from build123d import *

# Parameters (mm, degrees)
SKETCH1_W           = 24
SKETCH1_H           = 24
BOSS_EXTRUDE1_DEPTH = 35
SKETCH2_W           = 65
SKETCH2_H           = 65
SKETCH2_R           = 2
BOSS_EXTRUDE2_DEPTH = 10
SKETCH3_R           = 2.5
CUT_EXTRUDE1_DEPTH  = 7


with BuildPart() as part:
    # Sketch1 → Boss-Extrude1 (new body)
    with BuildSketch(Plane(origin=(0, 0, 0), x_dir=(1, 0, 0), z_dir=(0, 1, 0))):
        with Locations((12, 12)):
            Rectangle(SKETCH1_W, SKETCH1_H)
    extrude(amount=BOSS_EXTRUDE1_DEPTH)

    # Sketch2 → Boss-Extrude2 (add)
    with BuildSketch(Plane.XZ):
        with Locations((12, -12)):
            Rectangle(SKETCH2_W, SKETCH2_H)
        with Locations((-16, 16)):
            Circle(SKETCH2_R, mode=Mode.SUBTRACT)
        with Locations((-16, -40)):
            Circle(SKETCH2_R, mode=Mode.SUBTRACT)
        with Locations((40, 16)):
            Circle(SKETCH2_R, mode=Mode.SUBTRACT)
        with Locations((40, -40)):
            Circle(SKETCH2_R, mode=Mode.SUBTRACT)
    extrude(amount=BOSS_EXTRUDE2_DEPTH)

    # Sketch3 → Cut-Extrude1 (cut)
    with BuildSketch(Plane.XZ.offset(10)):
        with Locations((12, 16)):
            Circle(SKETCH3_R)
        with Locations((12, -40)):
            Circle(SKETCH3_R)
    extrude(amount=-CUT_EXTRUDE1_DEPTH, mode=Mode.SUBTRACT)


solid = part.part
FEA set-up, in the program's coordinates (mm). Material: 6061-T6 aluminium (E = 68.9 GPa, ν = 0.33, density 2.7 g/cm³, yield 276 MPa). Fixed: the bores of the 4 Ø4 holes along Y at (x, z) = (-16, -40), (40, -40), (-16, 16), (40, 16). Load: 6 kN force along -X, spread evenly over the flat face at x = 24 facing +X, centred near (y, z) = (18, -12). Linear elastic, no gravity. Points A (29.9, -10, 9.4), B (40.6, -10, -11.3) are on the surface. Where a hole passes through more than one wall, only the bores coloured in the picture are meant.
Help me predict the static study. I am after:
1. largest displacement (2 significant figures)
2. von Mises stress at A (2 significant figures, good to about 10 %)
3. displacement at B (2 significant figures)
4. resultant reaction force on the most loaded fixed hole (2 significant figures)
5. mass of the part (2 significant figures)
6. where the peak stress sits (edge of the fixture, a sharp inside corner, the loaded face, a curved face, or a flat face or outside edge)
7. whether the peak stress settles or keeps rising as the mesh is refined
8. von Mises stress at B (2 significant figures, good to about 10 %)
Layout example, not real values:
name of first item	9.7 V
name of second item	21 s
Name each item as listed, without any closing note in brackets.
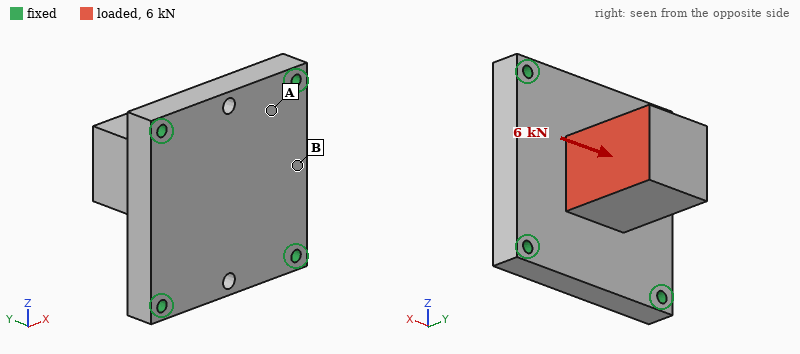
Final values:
largest displacement	94 µm
von Mises stress at A	9.9 MPa
displacement at B	20 µm
resultant reaction force on the most loaded fixed hole	2.2 kN
mass of the part	170 g
where the peak stress sits	edge of the fixture
whether the peak stress settles or keeps rising as the mesh is refined	keeps rising
von Mises stress at B	29 MPa
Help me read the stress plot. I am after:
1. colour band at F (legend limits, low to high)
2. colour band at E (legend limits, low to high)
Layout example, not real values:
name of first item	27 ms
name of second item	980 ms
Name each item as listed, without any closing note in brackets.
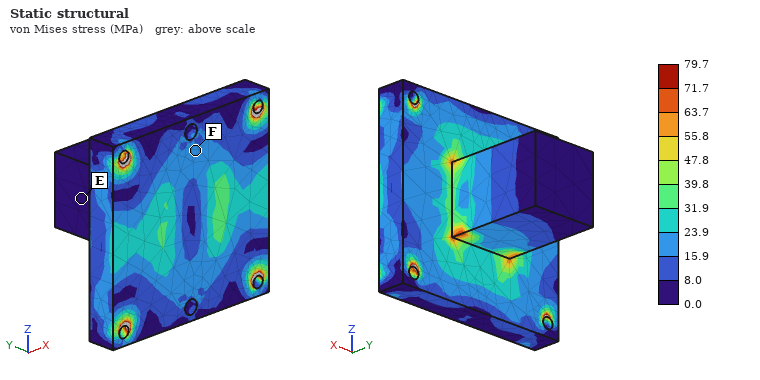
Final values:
colour band at F	15.9 to 23.9 MPa
colour band at E	0.0 to 8.0 MPa
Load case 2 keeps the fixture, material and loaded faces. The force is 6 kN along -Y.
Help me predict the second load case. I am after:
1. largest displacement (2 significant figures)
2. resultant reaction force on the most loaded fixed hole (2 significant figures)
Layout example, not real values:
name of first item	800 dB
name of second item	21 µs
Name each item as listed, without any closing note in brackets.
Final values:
largest displacement	74 µm
resultant reaction force on the most loaded fixed hole	2.2 kN
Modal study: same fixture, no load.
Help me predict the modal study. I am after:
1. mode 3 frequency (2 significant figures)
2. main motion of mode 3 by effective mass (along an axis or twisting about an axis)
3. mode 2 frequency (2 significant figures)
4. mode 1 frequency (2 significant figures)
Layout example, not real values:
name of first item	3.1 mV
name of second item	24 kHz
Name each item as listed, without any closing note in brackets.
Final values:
mode 3 frequency	6700 Hz
main motion of mode 3 by effective mass	along Y
mode 2 frequency	6300 Hz
mode 1 frequency	6300 Hz
